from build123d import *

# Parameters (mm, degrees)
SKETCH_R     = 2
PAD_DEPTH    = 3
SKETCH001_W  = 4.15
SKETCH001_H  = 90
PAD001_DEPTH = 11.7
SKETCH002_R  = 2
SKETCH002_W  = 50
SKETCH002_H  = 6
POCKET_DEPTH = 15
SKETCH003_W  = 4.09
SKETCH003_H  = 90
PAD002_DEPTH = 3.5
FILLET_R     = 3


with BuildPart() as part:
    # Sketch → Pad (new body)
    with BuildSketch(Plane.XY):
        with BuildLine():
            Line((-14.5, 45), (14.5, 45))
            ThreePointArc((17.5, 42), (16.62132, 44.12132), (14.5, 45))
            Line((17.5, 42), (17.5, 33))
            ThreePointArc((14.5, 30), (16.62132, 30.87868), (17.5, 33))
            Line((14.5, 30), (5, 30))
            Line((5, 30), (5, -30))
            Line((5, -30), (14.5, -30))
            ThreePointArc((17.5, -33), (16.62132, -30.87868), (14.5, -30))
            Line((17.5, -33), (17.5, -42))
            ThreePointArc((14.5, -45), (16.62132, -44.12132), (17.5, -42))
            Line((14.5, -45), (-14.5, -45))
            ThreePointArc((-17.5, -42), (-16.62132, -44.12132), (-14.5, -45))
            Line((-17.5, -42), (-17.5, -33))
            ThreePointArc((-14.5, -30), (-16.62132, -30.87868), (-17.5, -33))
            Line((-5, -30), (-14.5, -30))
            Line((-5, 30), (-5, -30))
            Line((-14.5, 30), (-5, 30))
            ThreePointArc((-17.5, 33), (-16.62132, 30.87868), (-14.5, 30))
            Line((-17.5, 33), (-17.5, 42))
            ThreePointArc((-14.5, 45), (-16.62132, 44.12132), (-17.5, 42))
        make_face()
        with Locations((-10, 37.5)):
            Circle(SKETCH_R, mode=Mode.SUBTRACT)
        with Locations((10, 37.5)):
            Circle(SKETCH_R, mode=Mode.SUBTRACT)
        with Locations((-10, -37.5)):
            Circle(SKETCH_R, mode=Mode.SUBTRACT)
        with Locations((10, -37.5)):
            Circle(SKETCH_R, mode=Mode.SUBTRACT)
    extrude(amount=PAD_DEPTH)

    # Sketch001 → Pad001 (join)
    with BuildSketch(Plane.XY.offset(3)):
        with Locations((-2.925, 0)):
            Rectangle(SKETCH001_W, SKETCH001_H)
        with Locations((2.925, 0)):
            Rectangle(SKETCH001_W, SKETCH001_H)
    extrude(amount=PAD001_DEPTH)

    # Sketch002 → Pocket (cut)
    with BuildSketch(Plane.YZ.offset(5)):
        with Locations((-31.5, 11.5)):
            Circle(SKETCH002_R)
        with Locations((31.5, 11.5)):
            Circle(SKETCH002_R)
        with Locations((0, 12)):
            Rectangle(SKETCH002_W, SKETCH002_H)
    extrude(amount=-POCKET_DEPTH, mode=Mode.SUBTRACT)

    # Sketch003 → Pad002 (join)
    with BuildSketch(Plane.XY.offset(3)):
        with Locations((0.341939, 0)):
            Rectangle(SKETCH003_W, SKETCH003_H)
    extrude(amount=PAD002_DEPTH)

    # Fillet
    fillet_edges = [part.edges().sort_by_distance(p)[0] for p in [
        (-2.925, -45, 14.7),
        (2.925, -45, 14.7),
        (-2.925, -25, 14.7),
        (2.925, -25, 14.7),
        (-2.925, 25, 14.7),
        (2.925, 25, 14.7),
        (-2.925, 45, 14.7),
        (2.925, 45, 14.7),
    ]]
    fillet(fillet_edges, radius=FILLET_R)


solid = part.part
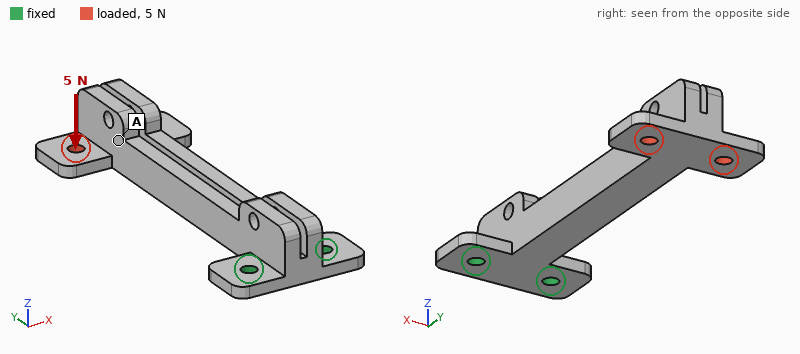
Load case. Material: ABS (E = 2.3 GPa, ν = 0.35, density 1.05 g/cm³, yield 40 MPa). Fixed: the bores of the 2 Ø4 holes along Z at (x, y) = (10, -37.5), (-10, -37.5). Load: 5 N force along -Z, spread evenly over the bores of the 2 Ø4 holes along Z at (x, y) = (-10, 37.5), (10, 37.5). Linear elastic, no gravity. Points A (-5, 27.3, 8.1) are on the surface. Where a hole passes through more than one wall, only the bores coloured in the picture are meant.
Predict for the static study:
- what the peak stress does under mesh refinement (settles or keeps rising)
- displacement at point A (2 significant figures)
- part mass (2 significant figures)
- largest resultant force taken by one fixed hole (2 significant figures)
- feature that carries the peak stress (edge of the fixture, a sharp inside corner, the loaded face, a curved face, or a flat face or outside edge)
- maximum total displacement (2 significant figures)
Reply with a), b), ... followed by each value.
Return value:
a) keeps rising
b) 0.73 mm
c) 12 g
d) 5.9 N
e) edge of the fixture
f) 1.0 mm
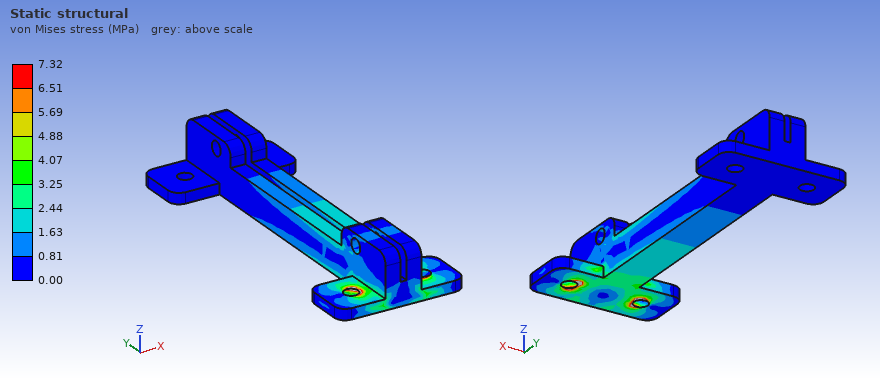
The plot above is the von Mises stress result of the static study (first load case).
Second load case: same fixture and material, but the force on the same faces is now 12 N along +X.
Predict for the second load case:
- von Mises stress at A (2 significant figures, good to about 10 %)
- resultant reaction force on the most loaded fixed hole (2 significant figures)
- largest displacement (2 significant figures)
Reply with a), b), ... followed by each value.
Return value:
a) 0.72 MPa
b) 45 N
c) 1.1 mm
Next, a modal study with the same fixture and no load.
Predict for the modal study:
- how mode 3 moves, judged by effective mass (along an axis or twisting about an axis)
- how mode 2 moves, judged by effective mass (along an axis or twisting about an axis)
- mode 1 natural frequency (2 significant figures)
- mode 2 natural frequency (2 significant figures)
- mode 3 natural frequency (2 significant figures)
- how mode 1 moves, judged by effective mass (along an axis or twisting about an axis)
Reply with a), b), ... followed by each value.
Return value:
a) twisting about Y
b) along X
c) 180 Hz
d) 280 Hz
e) 960 Hz
f) along Z
